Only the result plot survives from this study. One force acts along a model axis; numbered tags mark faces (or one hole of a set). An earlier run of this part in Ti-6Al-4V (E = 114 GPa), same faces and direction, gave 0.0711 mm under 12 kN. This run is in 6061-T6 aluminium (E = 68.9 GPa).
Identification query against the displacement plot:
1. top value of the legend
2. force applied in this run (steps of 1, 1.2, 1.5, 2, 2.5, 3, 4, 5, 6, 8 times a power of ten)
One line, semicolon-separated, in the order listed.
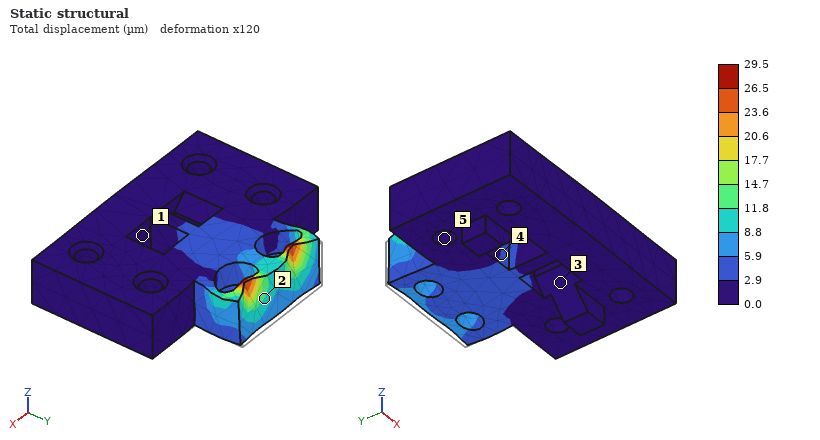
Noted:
29.5 µm; 3 kN
